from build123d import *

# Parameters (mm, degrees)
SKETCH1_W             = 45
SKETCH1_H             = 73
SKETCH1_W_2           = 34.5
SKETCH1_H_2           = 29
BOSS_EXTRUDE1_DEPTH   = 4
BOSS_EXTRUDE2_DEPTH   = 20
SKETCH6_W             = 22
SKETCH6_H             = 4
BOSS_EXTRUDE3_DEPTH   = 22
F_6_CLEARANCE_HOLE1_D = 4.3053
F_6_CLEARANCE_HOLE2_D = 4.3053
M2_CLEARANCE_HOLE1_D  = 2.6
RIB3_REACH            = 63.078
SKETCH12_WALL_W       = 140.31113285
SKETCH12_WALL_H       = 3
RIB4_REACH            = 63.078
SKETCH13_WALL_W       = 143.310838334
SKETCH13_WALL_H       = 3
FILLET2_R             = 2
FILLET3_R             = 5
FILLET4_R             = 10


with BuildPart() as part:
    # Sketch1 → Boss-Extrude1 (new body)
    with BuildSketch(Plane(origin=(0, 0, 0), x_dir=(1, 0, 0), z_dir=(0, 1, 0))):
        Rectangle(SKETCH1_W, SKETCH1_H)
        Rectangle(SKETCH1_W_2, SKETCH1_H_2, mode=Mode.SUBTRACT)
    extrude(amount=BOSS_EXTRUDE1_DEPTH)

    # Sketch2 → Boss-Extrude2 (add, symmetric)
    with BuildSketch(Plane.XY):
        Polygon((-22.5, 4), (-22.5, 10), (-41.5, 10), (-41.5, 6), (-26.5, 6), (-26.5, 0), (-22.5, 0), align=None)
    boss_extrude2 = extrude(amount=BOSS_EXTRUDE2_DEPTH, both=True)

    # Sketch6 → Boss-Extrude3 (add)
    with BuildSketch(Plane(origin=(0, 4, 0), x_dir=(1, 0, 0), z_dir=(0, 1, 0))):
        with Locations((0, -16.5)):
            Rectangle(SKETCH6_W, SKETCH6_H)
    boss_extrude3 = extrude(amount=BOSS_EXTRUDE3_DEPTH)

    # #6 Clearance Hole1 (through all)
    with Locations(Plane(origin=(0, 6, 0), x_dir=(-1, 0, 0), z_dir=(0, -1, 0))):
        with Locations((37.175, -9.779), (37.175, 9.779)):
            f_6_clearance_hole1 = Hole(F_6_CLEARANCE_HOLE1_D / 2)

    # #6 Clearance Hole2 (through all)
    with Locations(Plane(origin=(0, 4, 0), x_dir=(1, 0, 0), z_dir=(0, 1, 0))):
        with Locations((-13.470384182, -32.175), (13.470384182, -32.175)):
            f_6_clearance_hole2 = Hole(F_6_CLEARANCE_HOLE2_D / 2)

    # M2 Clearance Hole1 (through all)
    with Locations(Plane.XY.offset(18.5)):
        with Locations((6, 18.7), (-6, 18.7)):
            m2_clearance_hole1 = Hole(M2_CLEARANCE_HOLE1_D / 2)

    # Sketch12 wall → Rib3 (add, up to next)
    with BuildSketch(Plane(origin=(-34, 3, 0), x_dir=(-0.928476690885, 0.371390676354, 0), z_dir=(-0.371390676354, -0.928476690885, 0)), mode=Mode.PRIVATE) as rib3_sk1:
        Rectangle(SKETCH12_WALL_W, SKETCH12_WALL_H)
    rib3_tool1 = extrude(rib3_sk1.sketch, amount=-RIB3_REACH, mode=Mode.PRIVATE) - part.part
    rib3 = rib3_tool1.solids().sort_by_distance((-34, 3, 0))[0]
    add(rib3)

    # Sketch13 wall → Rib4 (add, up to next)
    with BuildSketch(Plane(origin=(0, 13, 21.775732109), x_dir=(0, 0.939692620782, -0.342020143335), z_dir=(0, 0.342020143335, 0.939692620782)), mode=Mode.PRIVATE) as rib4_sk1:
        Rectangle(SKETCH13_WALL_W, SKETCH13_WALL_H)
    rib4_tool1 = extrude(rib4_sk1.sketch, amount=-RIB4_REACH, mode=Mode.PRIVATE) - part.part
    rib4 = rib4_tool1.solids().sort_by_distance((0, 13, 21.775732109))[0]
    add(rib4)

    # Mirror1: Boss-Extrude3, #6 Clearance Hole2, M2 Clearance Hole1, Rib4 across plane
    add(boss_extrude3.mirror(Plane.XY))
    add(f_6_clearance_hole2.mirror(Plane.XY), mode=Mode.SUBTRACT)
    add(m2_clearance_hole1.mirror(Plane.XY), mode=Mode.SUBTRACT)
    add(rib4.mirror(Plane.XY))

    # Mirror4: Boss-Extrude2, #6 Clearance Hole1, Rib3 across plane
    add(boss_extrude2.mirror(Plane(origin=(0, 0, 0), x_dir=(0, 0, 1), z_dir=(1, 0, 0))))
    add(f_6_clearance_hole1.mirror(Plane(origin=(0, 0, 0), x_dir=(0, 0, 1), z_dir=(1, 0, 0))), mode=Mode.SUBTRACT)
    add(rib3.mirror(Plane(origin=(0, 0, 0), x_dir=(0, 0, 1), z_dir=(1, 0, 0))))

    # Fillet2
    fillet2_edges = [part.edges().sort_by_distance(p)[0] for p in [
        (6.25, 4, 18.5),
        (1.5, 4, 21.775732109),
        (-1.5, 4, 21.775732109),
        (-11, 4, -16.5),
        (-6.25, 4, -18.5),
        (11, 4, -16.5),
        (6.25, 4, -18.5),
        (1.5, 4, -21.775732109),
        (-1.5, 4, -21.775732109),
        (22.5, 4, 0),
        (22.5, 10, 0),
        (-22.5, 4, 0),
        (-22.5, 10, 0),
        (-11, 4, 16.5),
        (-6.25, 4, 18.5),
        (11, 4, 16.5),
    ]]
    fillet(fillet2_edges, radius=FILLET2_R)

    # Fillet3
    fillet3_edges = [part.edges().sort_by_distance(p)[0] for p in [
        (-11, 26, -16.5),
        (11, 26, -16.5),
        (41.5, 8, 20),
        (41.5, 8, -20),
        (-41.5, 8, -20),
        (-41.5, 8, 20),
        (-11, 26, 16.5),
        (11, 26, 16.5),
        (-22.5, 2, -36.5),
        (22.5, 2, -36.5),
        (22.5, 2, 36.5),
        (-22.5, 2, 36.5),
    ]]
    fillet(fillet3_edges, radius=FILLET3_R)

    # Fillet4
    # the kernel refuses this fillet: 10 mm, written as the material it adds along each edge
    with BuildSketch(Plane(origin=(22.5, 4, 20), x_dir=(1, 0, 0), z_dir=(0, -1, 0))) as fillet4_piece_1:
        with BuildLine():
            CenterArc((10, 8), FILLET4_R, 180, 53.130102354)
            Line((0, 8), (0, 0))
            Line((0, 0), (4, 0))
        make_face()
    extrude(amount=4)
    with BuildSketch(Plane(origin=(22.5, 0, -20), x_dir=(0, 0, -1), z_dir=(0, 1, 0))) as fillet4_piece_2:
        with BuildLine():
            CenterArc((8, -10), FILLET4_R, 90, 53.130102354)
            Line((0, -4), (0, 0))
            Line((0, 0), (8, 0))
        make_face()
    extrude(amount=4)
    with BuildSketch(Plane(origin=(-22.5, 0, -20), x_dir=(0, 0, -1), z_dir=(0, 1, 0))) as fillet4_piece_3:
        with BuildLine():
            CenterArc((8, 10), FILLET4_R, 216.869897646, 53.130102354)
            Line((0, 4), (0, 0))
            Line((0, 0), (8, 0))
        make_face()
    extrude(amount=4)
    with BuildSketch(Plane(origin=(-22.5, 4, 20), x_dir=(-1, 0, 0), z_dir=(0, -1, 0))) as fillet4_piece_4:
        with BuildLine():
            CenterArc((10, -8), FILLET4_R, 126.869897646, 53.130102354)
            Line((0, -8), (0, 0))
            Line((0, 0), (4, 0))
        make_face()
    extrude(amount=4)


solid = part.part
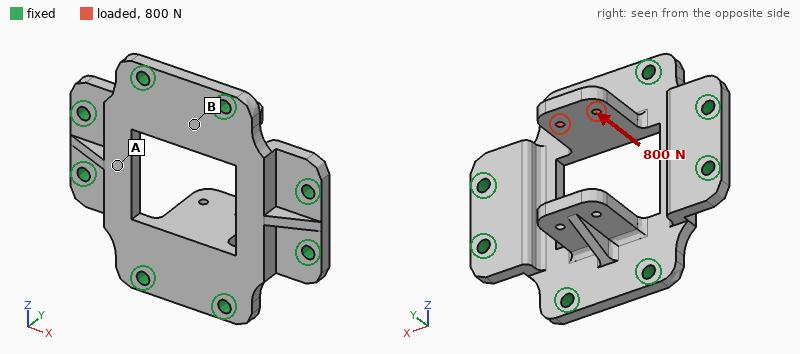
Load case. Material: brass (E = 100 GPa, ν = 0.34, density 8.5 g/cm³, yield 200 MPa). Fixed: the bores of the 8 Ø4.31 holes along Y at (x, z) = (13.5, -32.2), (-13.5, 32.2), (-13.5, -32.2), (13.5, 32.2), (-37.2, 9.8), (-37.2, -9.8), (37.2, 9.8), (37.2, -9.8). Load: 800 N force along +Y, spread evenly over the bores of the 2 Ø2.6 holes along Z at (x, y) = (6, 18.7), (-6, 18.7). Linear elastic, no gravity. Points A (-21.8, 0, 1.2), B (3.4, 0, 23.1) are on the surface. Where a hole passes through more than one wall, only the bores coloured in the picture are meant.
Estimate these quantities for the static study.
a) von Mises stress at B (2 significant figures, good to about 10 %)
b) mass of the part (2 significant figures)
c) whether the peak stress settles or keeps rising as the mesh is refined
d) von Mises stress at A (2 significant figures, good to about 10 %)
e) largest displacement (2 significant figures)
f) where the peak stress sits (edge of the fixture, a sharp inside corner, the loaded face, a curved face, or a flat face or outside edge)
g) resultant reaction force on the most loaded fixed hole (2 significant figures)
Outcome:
22 MPa
180 g
keeps rising
8.5 MPa
57 µm
edge of the fixture
290 N
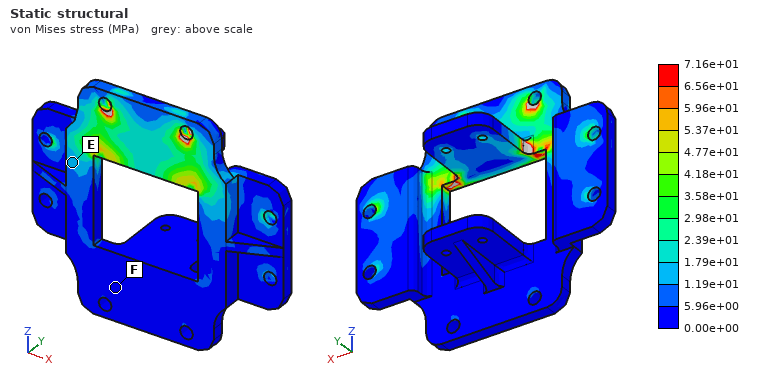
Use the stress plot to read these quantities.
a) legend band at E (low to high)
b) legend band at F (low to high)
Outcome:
1.19e+01 to 1.79e+01 MPa
0.00e+00 to 5.96e+00 MPa
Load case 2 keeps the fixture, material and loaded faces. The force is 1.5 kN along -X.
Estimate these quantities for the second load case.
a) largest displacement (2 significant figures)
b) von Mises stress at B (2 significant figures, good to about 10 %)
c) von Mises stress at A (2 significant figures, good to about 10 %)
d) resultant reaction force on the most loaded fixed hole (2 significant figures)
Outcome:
84 µm
39 MPa
14 MPa
1.2 kN
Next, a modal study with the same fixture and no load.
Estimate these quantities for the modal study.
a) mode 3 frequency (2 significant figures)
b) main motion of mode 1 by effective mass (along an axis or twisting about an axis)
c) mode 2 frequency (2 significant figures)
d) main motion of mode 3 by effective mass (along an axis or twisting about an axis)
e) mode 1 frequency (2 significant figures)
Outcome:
6000 Hz
along Y
3700 Hz
along X
3500 Hz
